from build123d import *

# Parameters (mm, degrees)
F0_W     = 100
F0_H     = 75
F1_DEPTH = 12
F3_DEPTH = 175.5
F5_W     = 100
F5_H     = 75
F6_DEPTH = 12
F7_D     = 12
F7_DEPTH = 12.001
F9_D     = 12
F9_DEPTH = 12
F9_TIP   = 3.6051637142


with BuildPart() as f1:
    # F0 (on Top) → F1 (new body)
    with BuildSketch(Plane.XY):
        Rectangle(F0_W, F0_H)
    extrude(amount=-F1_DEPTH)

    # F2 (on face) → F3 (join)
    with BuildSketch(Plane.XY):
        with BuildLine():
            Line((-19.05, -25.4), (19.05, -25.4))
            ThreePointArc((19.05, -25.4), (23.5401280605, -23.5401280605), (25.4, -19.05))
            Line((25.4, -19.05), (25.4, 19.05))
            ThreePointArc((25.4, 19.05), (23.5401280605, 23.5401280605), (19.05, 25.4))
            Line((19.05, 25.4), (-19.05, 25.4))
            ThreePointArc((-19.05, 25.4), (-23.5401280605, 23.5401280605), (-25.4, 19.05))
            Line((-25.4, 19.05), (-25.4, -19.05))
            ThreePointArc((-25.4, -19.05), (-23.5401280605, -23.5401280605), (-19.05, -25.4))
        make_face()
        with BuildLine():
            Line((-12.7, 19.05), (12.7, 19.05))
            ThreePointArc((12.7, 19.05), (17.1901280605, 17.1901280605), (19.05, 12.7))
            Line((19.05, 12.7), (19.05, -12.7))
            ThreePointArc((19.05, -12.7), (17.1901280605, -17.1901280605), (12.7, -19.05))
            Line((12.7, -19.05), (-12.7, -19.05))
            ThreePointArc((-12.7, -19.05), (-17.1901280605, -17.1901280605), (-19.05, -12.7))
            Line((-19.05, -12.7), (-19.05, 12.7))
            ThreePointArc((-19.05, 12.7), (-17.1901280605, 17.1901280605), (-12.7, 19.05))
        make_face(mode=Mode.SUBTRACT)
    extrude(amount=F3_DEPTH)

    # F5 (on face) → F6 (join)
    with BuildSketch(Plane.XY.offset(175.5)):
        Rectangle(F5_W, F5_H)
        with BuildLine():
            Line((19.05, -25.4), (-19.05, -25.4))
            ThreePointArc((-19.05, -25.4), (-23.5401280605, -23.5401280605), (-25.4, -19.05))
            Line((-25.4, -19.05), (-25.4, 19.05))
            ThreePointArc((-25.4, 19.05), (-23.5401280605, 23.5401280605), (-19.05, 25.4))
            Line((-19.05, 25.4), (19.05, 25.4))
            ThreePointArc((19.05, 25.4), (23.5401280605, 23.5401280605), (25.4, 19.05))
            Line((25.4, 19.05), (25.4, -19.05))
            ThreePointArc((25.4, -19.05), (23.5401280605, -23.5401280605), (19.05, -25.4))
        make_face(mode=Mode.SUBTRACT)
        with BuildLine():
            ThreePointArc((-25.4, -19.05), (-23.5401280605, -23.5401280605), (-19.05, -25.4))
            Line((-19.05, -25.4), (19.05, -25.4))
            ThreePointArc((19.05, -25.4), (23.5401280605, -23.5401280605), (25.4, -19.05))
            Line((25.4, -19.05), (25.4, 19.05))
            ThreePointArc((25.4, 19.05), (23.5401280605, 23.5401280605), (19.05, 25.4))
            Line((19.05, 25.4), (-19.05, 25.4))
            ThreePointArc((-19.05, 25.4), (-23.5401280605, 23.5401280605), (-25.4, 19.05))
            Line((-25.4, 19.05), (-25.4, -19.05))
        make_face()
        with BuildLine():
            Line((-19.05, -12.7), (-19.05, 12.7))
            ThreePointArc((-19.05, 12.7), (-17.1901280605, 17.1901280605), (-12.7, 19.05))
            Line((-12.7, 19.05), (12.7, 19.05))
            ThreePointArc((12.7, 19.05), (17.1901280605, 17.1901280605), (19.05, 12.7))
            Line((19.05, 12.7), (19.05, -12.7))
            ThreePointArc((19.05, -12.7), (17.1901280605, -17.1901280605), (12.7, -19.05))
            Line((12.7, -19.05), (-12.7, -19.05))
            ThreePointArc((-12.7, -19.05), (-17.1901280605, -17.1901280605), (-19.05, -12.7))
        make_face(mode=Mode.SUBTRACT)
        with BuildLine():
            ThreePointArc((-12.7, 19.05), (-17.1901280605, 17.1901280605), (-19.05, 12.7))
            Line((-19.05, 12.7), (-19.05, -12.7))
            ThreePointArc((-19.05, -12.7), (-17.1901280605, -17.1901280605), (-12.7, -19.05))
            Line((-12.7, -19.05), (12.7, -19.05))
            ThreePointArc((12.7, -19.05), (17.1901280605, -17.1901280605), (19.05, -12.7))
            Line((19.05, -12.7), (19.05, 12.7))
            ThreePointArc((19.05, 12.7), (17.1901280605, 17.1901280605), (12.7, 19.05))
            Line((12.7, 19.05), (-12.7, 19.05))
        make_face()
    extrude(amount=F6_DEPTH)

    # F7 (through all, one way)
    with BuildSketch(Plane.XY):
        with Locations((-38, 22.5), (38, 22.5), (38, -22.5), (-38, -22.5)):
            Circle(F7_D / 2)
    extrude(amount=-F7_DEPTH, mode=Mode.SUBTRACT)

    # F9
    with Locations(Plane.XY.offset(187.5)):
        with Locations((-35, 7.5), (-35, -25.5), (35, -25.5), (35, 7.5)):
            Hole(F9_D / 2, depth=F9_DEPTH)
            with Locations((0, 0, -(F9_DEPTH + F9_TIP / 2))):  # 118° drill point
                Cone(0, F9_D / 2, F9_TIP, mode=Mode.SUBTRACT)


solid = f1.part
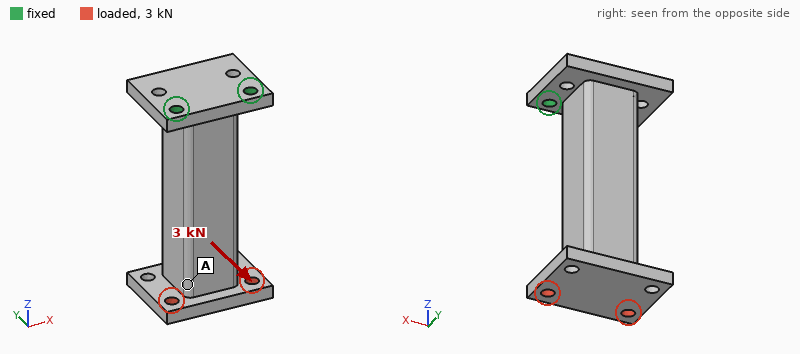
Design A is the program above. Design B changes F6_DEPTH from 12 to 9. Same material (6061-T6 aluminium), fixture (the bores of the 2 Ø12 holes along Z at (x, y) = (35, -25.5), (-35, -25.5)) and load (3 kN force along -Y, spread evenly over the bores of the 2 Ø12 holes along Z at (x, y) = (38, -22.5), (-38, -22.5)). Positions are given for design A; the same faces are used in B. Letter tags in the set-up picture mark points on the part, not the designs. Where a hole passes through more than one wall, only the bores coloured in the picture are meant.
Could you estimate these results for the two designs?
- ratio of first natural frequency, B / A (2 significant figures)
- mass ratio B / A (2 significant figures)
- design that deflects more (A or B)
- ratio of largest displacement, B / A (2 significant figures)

0.76
0.94
B
1.7
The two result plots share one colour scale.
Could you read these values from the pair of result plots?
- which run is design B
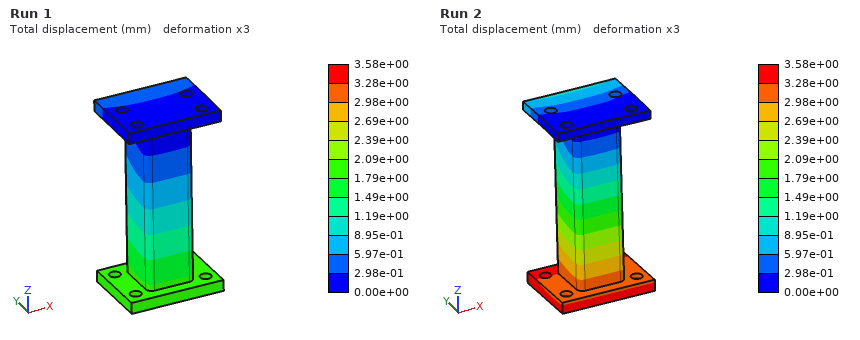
Run 2
